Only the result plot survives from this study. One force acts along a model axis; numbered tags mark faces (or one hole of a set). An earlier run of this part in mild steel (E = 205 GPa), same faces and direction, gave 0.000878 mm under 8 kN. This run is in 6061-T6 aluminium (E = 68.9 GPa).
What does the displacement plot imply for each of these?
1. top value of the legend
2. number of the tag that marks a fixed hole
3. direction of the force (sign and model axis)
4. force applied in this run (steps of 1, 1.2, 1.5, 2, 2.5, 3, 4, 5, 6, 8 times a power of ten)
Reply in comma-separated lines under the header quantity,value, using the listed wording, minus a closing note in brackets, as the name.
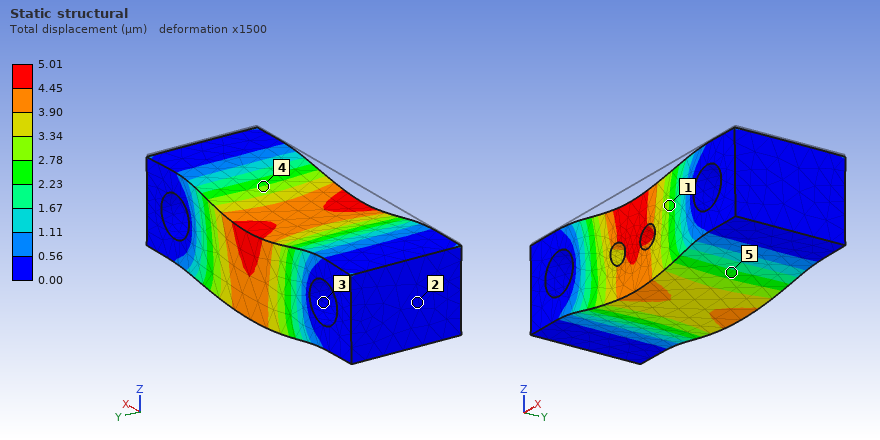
quantity,value
top value of the legend,5.01 µm
number of the tag that marks a fixed hole,3
direction of the force,-Z
force applied in this run,15 kN
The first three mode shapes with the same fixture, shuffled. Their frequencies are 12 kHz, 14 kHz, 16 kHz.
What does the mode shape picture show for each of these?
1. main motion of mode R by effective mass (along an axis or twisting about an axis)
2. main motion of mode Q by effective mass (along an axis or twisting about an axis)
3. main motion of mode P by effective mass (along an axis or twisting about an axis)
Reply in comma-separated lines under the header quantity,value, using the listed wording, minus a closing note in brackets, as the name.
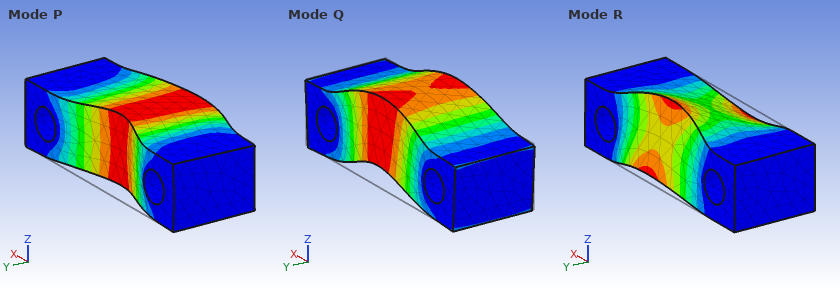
quantity,value
main motion of mode R by effective mass,twisting about X
main motion of mode Q by effective mass,along Z
main motion of mode P by effective mass,along Y
